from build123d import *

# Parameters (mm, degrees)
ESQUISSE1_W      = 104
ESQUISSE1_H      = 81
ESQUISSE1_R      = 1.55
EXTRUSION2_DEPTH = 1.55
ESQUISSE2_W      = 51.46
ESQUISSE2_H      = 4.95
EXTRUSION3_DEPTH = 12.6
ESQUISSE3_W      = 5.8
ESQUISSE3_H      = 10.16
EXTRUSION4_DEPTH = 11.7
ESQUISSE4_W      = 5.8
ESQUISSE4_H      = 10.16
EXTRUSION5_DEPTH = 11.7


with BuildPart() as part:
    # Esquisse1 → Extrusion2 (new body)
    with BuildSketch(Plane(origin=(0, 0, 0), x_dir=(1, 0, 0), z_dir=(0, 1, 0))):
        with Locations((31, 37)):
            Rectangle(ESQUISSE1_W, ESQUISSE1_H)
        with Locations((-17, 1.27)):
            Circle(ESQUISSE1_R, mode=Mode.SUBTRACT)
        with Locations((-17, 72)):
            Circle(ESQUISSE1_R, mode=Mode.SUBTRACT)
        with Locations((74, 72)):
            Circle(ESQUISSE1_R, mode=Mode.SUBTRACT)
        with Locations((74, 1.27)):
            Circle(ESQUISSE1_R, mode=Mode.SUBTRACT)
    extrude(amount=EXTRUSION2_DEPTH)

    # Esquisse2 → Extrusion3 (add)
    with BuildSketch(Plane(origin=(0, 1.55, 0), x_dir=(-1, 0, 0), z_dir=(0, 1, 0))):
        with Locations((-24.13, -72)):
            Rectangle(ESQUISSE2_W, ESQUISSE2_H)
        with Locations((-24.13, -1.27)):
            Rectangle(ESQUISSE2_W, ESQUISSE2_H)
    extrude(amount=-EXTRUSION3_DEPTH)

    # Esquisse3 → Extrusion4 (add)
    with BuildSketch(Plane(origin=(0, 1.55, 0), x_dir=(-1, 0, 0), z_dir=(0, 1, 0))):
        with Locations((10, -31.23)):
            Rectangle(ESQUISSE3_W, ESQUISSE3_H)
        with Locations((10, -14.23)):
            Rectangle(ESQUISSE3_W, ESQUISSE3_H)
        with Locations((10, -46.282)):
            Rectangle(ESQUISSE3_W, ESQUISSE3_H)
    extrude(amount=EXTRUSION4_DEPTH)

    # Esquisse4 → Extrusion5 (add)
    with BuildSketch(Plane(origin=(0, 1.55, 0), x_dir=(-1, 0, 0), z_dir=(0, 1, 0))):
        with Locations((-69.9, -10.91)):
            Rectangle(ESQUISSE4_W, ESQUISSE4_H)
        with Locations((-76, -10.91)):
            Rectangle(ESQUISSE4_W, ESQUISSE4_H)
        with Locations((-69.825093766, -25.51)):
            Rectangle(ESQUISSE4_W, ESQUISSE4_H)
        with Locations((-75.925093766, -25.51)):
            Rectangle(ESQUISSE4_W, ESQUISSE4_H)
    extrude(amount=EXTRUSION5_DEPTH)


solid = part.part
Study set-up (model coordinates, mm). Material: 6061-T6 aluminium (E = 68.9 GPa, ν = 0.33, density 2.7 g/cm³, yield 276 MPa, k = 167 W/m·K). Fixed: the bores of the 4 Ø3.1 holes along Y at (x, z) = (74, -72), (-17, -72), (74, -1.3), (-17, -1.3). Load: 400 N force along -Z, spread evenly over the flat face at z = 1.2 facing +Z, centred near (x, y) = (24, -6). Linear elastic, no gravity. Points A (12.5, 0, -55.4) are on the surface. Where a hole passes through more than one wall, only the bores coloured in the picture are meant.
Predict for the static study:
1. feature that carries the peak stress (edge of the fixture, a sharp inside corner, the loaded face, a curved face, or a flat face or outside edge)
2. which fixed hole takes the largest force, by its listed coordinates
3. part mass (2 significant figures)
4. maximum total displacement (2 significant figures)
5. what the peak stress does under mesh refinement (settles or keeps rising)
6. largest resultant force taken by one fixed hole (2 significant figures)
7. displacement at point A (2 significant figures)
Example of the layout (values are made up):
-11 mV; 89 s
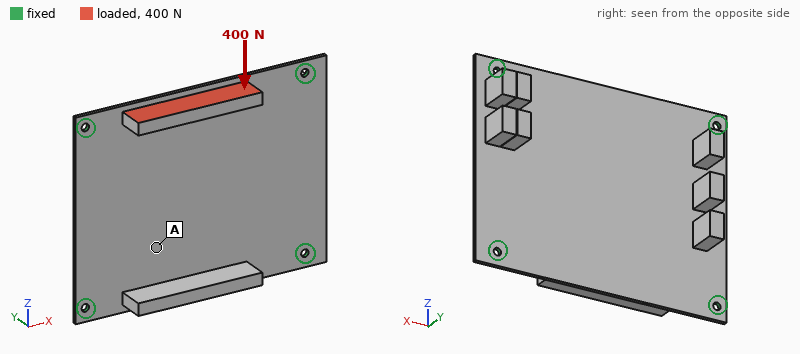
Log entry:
edge of the fixture; (-17, -1.3); 63 g; 0.26 mm; keeps rising; 140 N; 0.086 mm
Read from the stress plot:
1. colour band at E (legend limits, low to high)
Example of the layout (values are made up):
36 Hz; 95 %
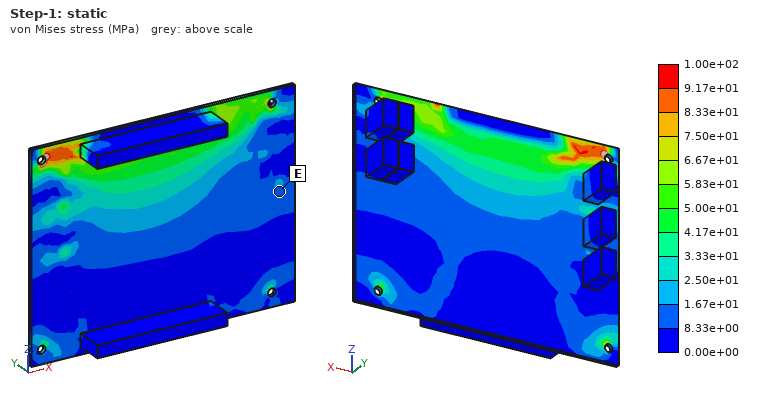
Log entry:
8.33e+00 to 1.67e+01 MPa
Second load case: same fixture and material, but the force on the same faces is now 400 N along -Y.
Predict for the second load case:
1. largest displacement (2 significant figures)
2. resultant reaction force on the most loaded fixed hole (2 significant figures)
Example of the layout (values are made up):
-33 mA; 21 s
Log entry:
0.63 mm; 300 N
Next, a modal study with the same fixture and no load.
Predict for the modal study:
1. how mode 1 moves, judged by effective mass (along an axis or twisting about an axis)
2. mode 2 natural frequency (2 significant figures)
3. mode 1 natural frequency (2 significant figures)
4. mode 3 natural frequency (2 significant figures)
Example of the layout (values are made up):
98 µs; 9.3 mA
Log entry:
along Y; 1300 Hz; 910 Hz; 1400 Hz
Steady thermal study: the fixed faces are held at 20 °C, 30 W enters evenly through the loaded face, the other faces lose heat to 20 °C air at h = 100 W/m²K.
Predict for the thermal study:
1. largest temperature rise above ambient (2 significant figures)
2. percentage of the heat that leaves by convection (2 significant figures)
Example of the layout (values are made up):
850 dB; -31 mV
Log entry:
37 K; 65 %
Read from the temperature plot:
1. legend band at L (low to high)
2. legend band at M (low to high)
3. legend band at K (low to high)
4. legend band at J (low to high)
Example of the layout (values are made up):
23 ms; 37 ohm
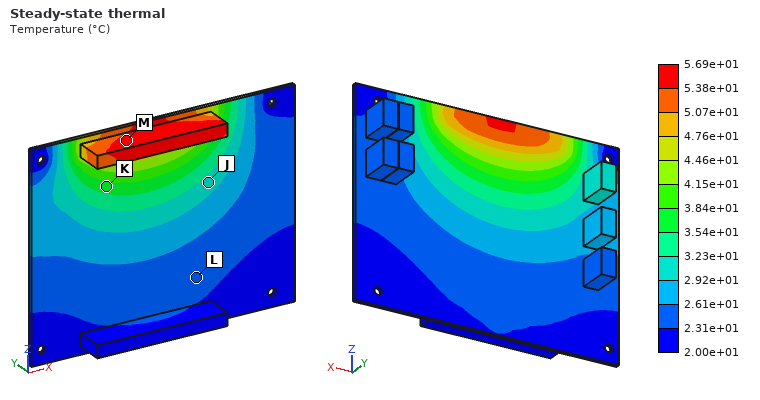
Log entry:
2.31e+01 to 2.61e+01 °C; 5.38e+01 to 5.69e+01 °C; 3.54e+01 to 3.84e+01 °C; 2.92e+01 to 3.23e+01 °C
